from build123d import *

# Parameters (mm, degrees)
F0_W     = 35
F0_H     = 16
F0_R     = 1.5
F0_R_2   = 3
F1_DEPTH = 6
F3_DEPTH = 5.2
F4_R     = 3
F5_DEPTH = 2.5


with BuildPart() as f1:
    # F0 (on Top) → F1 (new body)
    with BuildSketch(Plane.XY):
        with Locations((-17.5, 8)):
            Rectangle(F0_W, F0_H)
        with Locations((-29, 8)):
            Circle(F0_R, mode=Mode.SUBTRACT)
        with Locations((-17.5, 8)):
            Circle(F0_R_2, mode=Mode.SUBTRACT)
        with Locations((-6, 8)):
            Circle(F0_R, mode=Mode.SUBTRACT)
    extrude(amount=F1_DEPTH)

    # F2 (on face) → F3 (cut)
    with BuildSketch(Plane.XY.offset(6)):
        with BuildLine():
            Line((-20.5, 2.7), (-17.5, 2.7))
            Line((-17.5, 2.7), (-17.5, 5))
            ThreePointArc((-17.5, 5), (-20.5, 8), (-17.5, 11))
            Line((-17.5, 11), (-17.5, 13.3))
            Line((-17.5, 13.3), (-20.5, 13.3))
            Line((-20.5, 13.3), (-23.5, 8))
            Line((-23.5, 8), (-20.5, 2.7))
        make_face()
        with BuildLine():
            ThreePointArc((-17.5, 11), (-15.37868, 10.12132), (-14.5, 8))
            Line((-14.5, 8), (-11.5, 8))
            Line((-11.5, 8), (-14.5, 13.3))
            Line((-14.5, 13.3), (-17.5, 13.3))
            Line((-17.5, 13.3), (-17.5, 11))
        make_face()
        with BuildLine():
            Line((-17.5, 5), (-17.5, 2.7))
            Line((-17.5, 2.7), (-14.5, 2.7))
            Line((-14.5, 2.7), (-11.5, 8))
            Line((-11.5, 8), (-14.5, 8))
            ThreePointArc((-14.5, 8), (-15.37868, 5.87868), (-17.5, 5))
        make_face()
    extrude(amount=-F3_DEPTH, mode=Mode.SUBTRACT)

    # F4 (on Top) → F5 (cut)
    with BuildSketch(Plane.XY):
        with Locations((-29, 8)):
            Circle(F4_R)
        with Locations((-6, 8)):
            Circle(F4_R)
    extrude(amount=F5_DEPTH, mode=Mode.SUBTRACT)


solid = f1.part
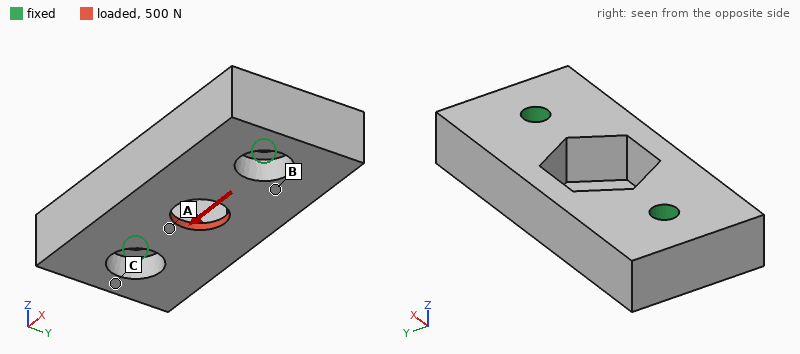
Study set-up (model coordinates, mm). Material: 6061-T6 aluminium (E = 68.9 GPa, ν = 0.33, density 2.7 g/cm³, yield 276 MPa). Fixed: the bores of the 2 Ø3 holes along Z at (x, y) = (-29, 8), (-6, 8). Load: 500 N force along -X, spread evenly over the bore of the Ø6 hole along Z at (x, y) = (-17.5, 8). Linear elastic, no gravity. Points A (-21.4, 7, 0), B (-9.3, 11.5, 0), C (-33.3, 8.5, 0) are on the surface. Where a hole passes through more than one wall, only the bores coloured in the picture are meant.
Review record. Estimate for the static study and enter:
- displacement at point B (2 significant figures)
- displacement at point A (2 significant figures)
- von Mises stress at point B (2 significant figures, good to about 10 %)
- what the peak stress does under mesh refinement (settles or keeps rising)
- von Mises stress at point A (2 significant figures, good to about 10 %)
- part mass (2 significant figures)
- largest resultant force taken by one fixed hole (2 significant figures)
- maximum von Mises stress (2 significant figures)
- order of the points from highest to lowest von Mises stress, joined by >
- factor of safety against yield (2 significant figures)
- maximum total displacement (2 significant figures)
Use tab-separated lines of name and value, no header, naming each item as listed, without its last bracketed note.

displacement at point B	1.2 µm
displacement at point A	3.2 µm
von Mises stress at point B	11 MPa
what the peak stress does under mesh refinement	settles
von Mises stress at point A	33 MPa
part mass	7.2 g
largest resultant force taken by one fixed hole	260 N
maximum von Mises stress	60 MPa
order of the points from highest to lowest von Mises stress, joined by >	A > B > C
factor of safety against yield	4.6
maximum total displacement	3.9 µm
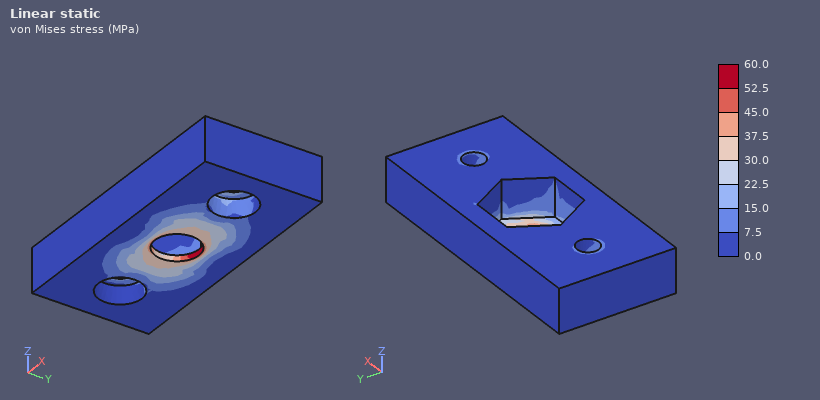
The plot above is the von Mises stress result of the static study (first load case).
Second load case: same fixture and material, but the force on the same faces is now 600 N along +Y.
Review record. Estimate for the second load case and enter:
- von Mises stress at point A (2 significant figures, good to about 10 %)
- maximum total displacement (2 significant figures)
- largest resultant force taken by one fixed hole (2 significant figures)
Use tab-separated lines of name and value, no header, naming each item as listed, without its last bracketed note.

von Mises stress at point A	41 MPa
maximum total displacement	9.5 µm
largest resultant force taken by one fixed hole	300 N
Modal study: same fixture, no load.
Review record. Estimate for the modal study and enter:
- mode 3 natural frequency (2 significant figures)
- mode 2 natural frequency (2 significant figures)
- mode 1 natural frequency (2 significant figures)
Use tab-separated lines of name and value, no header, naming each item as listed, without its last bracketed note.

mode 3 natural frequency	32 kHz
mode 2 natural frequency	31 kHz
mode 1 natural frequency	23 kHz
